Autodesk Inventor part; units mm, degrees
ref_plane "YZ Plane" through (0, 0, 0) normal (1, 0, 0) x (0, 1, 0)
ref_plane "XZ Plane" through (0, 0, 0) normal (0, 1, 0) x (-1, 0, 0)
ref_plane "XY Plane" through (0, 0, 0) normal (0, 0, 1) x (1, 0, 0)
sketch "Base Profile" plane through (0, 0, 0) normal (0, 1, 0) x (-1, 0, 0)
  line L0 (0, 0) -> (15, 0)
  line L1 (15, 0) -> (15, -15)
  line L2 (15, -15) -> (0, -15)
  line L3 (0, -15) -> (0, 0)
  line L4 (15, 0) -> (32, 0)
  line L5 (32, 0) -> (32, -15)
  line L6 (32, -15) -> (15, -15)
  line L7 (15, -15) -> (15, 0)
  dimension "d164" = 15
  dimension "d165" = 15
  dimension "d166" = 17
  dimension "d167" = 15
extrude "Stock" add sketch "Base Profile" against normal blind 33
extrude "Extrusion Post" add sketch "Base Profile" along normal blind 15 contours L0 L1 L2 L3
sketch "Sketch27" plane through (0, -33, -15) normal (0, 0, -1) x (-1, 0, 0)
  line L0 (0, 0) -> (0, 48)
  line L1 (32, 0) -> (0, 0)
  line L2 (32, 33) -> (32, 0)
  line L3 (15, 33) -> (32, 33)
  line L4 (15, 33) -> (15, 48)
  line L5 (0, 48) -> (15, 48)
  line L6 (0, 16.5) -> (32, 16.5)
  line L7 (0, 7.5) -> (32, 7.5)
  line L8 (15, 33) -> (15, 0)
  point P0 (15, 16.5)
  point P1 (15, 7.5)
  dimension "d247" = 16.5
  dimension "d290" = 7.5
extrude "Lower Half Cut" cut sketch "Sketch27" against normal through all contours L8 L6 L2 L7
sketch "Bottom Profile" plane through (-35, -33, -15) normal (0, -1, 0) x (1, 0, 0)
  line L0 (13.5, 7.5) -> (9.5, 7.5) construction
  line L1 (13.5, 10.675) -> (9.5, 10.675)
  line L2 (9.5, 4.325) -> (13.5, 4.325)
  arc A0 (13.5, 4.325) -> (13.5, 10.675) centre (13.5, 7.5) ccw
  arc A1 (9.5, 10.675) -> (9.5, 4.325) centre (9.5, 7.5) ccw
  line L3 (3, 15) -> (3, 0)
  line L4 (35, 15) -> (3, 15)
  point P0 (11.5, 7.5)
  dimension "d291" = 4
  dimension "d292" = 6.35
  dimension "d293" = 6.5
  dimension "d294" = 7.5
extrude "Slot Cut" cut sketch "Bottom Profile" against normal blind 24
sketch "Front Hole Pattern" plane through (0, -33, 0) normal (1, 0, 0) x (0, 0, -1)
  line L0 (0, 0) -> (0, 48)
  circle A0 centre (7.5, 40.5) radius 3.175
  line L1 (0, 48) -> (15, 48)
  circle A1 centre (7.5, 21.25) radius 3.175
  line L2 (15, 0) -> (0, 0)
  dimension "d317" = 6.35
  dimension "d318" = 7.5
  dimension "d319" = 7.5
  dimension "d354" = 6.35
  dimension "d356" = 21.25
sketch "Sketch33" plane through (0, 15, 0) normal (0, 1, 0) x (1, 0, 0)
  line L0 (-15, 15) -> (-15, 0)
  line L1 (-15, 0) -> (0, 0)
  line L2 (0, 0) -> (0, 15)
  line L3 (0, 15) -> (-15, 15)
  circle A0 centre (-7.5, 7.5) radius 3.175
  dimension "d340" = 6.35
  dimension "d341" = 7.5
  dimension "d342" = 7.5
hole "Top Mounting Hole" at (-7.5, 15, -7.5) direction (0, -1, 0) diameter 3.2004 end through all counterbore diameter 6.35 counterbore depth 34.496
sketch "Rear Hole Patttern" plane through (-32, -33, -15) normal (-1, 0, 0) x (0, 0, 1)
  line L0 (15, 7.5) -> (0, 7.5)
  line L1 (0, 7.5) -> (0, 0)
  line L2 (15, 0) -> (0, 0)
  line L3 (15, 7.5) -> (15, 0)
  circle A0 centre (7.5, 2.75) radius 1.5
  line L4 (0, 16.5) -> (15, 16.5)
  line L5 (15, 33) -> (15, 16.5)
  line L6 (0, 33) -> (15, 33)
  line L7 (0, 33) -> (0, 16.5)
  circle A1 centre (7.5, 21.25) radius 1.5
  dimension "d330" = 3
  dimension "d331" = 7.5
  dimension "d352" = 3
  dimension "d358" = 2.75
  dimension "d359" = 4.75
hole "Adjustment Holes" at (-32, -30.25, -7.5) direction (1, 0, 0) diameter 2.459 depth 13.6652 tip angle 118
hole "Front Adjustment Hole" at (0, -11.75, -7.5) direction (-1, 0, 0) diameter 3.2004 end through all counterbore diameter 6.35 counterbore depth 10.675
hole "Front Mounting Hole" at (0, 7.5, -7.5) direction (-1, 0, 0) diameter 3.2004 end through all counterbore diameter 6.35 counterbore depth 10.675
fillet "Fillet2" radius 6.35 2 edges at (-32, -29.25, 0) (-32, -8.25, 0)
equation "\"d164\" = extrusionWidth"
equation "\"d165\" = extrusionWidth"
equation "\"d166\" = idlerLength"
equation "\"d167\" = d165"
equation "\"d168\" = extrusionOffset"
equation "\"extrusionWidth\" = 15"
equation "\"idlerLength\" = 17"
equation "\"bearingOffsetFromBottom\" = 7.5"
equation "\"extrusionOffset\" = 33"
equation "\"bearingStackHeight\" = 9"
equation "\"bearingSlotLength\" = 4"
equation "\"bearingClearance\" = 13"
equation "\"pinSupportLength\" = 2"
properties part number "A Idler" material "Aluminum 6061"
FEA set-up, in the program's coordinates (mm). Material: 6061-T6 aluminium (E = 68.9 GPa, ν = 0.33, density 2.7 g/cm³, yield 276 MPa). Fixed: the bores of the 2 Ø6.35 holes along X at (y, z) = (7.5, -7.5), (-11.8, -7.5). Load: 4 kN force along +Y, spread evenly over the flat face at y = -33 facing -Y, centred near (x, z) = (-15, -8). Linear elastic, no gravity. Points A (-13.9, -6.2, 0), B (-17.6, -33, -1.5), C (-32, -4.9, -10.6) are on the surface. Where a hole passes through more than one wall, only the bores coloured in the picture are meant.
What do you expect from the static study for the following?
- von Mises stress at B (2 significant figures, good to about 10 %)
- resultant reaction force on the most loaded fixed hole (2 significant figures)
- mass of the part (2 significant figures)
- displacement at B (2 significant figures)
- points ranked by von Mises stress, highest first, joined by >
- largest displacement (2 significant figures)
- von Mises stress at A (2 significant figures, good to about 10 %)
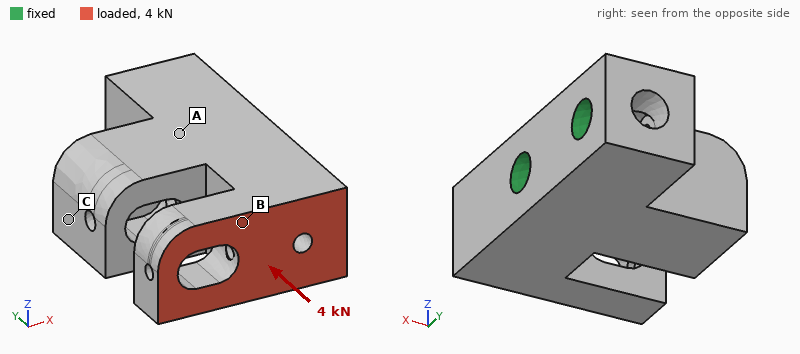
110 MPa
2.6 kN
38 g
0.068 mm
B > A > C
0.17 mm
30 MPa
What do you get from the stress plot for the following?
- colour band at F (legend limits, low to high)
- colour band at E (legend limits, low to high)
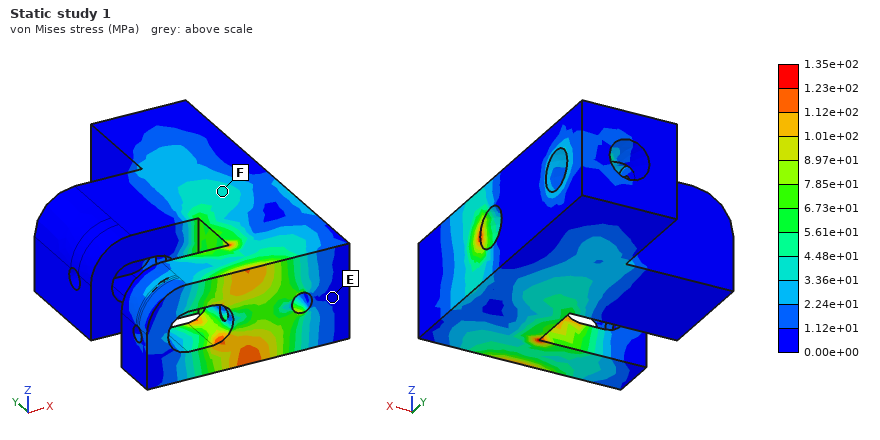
3.36e+01 to 4.48e+01 MPa
0.00e+00 to 1.12e+01 MPa
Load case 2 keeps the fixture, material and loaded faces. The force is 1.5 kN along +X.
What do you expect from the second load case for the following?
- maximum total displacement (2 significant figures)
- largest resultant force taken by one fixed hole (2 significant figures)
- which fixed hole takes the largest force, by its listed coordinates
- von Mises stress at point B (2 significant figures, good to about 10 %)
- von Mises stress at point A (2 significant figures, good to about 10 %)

72 µm
2.7 kN
(-11.8, -7.5)
28 MPa
20 MPa
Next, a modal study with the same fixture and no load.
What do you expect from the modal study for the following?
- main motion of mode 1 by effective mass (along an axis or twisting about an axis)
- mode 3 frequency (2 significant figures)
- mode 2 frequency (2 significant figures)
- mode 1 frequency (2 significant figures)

along Z
12 kHz
9300 Hz
7900 Hz
